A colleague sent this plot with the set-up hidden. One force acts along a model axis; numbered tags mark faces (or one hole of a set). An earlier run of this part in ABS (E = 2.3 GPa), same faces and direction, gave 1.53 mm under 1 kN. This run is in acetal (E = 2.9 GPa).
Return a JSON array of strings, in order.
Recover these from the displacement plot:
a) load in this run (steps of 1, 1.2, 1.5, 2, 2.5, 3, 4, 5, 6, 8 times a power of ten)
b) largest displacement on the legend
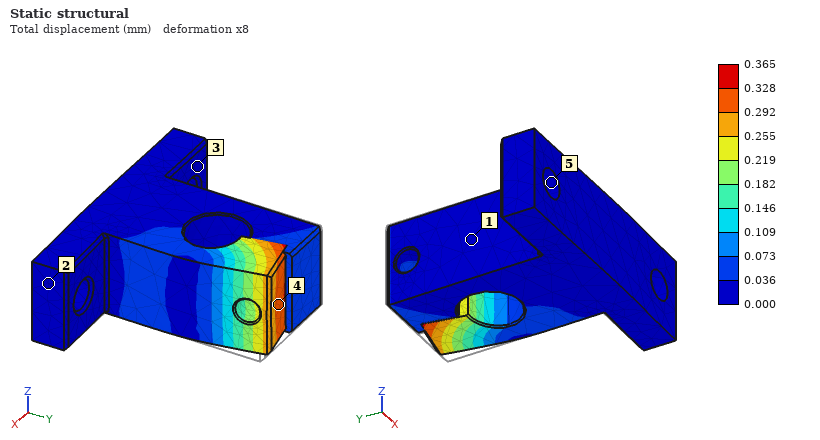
["300 N", "0.365 mm"]
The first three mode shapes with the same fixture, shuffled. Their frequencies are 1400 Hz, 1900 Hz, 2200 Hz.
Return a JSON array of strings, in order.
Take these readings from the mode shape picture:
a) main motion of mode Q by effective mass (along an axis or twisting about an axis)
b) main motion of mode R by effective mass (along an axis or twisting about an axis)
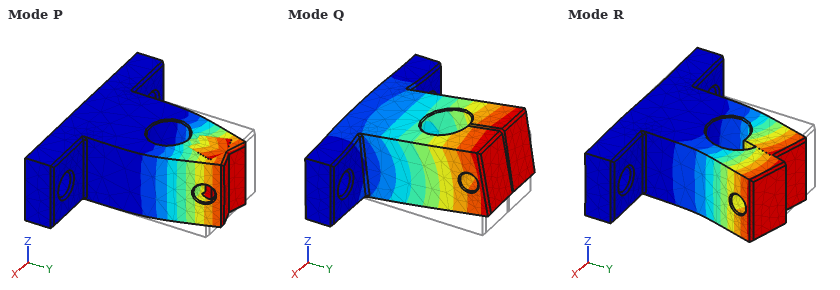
["along Z", "along X"]
